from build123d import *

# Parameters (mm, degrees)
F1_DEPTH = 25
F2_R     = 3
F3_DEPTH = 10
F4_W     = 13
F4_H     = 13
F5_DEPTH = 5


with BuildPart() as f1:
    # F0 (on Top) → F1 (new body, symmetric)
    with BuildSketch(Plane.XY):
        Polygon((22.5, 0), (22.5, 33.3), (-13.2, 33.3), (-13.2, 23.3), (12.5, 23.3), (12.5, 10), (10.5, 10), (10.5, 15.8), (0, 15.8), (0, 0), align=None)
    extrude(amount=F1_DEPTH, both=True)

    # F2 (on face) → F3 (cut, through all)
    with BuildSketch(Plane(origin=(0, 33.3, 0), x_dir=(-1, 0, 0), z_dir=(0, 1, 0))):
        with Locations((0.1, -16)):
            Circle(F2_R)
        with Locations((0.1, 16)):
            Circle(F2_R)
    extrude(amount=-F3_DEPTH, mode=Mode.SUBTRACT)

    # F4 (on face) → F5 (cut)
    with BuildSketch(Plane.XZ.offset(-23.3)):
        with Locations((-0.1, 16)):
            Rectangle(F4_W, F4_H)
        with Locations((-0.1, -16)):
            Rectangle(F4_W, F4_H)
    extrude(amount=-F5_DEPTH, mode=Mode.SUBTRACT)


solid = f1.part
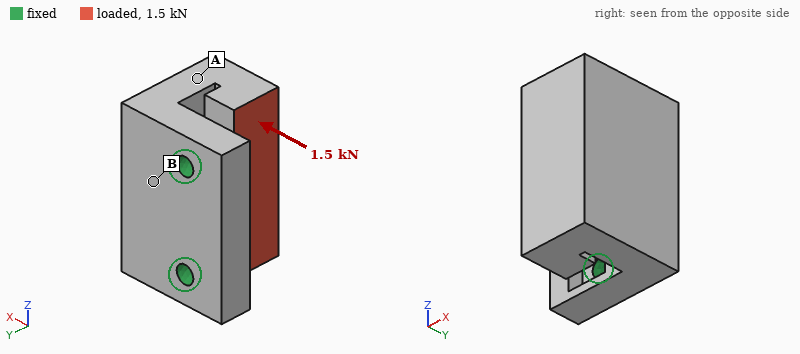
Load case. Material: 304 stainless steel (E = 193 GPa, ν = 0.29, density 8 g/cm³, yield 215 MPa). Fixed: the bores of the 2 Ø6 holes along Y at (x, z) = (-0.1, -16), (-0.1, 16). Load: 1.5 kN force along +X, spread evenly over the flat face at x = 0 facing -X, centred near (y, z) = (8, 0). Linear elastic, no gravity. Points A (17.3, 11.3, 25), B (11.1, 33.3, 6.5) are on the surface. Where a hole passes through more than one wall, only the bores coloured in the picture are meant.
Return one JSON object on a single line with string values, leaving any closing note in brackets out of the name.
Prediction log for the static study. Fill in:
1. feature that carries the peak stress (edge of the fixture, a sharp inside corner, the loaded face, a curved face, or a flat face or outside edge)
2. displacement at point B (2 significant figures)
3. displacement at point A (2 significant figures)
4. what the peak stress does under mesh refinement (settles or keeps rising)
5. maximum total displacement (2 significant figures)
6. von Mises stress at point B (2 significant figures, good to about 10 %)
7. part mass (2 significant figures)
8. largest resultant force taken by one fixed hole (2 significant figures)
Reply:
{"feature that carries the peak stress": "edge of the fixture", "displacement at point B": "11 µm", "displacement at point A": "36 µm", "what the peak stress does under mesh refinement": "keeps rising", "maximum total displacement": "59 µm", "von Mises stress at point B": "35 MPa", "part mass": "290 g", "largest resultant force taken by one fixed hole": "750 N"}
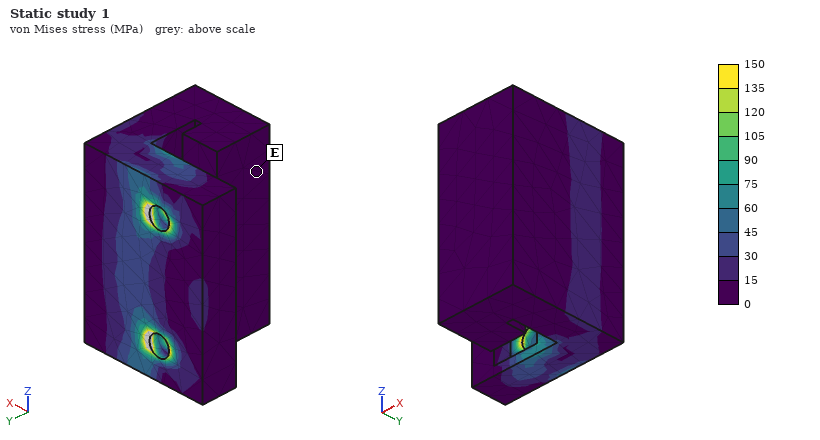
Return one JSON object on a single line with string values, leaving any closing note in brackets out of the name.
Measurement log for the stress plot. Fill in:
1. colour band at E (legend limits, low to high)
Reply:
{"colour band at E": "0 to 15 MPa"}
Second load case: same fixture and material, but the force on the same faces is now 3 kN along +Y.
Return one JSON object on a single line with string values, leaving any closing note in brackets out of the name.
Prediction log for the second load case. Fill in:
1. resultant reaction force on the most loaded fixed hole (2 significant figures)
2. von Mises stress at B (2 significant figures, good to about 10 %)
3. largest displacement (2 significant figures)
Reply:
{"resultant reaction force on the most loaded fixed hole": "1.5 kN", "von Mises stress at B": "36 MPa", "largest displacement": "52 µm"}
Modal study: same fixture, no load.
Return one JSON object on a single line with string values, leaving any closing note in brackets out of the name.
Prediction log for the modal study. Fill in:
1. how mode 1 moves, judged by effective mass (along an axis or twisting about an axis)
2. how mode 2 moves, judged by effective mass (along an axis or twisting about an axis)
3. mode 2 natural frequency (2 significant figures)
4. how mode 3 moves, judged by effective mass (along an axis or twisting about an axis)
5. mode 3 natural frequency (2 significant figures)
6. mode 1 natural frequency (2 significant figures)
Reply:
{"how mode 1 moves, judged by effective mass": "along X", "how mode 2 moves, judged by effective mass": "along Z", "mode 2 natural frequency": "4400 Hz", "how mode 3 moves, judged by effective mass": "along Y", "mode 3 natural frequency": "6500 Hz", "mode 1 natural frequency": "2300 Hz"}
